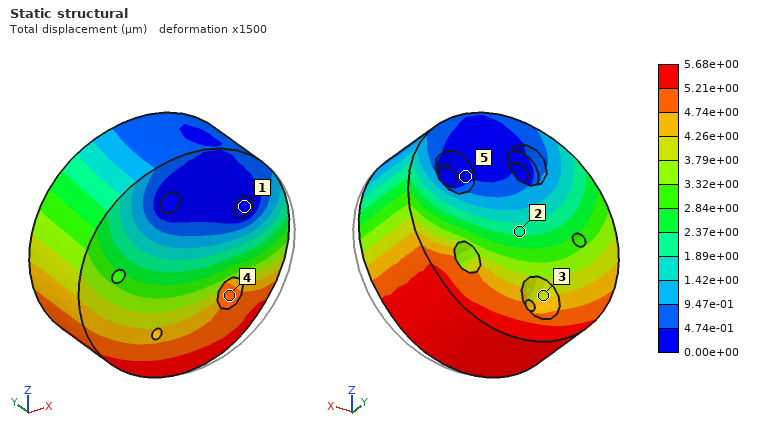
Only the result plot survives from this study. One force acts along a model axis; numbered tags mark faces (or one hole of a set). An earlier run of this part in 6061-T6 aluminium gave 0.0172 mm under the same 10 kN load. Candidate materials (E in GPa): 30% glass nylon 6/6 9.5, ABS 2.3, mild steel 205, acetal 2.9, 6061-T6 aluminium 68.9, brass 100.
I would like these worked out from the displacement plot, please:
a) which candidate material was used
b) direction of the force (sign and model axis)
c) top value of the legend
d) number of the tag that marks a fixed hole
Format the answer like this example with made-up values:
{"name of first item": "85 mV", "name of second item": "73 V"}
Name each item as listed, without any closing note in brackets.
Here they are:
{"which candidate material was used": "mild steel", "direction of the force": "-X", "top value of the legend": "5.68e+00 µm", "number of the tag that marks a fixed hole": "1"}
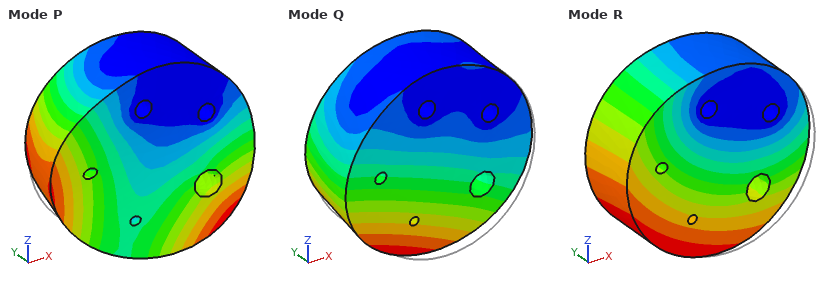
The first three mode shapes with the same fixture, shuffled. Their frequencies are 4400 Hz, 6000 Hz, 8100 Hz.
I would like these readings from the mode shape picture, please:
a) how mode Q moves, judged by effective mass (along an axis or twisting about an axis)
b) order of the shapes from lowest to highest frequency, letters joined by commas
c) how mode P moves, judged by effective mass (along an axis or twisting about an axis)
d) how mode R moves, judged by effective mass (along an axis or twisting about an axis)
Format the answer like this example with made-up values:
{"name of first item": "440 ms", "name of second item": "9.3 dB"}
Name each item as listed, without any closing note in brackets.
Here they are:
{"how mode Q moves, judged by effective mass": "along Y", "order of the shapes from lowest to highest frequency, letters joined by commas": "Q, R, P", "how mode P moves, judged by effective mass": "twisting about Z", "how mode R moves, judged by effective mass": "along X"}
